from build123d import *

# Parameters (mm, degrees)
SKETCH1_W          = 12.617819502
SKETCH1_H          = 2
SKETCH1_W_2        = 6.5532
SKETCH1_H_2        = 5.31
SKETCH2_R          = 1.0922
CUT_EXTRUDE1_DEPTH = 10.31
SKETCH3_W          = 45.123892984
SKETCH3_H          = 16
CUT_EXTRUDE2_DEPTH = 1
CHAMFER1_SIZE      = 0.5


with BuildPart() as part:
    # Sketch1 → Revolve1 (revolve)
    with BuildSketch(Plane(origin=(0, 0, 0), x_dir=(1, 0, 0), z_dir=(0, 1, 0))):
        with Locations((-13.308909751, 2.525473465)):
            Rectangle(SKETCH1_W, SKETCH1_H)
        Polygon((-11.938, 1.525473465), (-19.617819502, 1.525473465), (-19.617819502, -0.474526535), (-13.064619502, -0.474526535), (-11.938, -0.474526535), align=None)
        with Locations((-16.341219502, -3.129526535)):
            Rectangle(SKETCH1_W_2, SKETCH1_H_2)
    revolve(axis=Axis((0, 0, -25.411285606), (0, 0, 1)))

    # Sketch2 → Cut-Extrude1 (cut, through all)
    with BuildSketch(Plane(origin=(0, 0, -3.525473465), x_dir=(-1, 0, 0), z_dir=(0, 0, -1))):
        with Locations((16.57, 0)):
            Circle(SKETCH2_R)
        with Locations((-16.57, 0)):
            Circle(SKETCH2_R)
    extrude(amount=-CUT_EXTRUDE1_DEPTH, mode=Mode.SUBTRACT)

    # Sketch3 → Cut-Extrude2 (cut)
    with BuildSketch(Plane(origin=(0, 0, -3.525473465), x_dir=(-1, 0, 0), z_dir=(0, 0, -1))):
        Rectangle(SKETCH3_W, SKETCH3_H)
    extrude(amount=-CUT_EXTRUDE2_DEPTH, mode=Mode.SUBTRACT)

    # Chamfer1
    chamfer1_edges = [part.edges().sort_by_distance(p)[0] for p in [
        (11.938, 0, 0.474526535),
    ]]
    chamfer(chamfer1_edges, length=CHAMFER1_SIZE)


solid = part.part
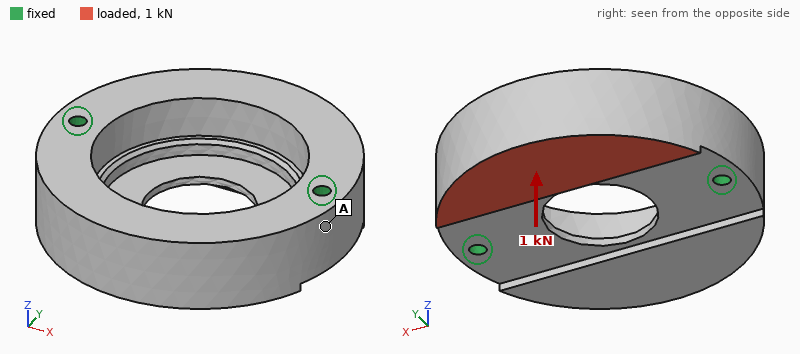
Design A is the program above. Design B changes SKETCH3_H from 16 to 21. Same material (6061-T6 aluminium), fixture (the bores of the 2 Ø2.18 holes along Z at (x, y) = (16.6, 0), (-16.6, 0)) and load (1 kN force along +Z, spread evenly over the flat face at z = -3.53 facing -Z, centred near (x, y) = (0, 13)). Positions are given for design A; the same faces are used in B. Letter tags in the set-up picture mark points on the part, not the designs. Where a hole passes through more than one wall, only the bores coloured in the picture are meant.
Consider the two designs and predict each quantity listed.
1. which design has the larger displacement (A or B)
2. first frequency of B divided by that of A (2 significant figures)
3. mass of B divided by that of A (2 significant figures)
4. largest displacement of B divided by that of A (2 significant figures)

B
1.0
0.97
1.2
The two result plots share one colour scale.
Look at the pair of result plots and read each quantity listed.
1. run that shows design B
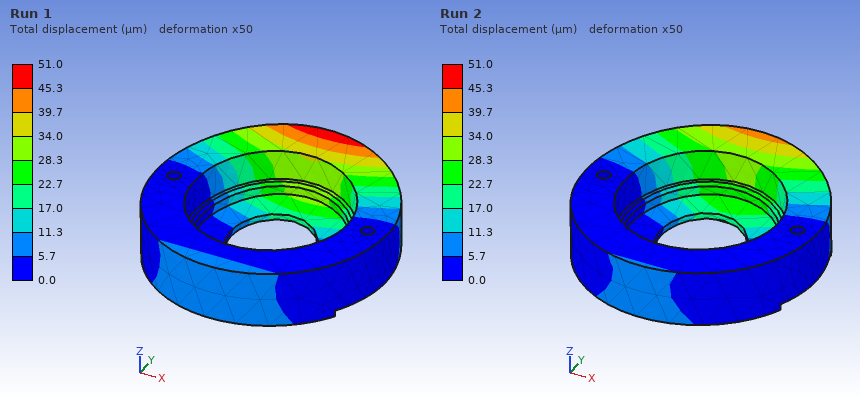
Run 1
